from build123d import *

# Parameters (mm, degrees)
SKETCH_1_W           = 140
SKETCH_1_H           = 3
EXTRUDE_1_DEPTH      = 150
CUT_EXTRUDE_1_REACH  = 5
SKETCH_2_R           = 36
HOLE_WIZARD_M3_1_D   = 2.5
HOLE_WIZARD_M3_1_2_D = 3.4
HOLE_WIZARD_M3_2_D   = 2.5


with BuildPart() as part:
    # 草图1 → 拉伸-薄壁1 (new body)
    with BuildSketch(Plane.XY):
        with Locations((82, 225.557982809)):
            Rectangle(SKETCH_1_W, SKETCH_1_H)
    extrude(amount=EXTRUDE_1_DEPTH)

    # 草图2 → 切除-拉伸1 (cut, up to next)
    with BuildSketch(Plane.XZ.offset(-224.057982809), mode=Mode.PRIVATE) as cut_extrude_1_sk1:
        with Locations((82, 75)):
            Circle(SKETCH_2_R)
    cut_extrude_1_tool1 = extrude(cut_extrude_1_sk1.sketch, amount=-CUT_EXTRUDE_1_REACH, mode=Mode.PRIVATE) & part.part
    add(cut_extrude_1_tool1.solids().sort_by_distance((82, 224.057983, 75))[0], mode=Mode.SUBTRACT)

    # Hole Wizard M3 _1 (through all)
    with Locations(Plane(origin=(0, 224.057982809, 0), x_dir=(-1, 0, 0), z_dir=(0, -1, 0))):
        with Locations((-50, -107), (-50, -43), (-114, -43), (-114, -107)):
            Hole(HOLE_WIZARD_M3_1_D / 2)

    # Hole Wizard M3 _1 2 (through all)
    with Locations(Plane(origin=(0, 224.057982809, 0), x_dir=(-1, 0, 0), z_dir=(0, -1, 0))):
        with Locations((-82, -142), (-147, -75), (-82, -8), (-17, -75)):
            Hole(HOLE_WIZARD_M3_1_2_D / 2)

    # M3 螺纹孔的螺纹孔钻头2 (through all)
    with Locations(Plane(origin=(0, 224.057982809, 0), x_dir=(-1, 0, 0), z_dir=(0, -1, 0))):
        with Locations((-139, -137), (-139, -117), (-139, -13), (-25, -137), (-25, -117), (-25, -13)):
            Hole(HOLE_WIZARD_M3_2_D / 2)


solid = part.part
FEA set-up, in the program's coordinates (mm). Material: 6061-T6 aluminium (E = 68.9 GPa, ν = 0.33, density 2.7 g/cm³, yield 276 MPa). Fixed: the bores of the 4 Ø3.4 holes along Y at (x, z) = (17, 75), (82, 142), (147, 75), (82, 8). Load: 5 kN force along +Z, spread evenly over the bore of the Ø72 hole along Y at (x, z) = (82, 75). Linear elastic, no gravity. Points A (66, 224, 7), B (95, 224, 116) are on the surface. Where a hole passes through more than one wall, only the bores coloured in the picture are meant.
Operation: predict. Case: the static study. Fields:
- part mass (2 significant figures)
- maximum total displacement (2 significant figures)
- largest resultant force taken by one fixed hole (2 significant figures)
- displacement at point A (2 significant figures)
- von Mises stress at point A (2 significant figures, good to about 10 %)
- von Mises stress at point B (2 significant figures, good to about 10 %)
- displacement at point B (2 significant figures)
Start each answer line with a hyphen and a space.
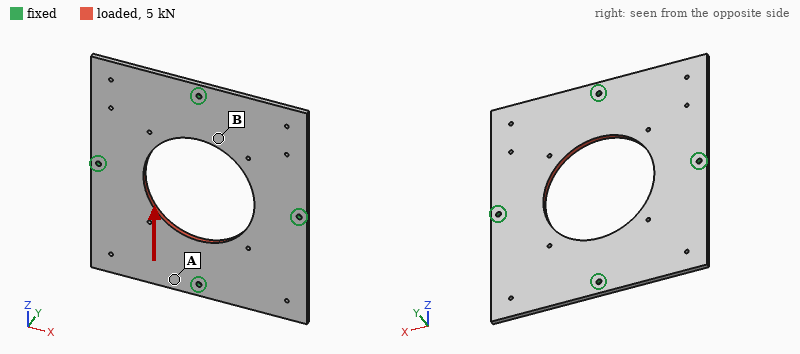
- 140 g
- 13 µm
- 1.3 kN
- 6.0 µm
- 4.5 MPa
- 12 MPa
- 8.2 µm
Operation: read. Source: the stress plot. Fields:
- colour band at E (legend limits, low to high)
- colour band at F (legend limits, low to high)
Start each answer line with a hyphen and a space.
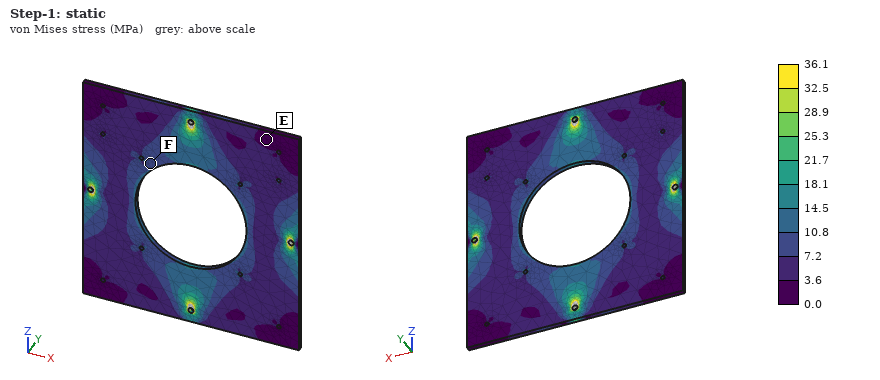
- 0.0 to 3.6 MPa
- 7.2 to 10.8 MPa
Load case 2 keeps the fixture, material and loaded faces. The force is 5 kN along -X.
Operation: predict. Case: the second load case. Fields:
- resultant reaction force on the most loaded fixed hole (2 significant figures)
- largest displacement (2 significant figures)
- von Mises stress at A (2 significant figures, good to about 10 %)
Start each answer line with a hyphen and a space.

- 1.3 kN
- 12 µm
- 9.7 MPa
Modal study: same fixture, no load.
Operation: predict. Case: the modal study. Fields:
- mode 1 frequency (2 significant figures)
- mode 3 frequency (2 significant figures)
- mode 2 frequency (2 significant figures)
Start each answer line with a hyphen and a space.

- 810 Hz
- 870 Hz
- 860 Hz
